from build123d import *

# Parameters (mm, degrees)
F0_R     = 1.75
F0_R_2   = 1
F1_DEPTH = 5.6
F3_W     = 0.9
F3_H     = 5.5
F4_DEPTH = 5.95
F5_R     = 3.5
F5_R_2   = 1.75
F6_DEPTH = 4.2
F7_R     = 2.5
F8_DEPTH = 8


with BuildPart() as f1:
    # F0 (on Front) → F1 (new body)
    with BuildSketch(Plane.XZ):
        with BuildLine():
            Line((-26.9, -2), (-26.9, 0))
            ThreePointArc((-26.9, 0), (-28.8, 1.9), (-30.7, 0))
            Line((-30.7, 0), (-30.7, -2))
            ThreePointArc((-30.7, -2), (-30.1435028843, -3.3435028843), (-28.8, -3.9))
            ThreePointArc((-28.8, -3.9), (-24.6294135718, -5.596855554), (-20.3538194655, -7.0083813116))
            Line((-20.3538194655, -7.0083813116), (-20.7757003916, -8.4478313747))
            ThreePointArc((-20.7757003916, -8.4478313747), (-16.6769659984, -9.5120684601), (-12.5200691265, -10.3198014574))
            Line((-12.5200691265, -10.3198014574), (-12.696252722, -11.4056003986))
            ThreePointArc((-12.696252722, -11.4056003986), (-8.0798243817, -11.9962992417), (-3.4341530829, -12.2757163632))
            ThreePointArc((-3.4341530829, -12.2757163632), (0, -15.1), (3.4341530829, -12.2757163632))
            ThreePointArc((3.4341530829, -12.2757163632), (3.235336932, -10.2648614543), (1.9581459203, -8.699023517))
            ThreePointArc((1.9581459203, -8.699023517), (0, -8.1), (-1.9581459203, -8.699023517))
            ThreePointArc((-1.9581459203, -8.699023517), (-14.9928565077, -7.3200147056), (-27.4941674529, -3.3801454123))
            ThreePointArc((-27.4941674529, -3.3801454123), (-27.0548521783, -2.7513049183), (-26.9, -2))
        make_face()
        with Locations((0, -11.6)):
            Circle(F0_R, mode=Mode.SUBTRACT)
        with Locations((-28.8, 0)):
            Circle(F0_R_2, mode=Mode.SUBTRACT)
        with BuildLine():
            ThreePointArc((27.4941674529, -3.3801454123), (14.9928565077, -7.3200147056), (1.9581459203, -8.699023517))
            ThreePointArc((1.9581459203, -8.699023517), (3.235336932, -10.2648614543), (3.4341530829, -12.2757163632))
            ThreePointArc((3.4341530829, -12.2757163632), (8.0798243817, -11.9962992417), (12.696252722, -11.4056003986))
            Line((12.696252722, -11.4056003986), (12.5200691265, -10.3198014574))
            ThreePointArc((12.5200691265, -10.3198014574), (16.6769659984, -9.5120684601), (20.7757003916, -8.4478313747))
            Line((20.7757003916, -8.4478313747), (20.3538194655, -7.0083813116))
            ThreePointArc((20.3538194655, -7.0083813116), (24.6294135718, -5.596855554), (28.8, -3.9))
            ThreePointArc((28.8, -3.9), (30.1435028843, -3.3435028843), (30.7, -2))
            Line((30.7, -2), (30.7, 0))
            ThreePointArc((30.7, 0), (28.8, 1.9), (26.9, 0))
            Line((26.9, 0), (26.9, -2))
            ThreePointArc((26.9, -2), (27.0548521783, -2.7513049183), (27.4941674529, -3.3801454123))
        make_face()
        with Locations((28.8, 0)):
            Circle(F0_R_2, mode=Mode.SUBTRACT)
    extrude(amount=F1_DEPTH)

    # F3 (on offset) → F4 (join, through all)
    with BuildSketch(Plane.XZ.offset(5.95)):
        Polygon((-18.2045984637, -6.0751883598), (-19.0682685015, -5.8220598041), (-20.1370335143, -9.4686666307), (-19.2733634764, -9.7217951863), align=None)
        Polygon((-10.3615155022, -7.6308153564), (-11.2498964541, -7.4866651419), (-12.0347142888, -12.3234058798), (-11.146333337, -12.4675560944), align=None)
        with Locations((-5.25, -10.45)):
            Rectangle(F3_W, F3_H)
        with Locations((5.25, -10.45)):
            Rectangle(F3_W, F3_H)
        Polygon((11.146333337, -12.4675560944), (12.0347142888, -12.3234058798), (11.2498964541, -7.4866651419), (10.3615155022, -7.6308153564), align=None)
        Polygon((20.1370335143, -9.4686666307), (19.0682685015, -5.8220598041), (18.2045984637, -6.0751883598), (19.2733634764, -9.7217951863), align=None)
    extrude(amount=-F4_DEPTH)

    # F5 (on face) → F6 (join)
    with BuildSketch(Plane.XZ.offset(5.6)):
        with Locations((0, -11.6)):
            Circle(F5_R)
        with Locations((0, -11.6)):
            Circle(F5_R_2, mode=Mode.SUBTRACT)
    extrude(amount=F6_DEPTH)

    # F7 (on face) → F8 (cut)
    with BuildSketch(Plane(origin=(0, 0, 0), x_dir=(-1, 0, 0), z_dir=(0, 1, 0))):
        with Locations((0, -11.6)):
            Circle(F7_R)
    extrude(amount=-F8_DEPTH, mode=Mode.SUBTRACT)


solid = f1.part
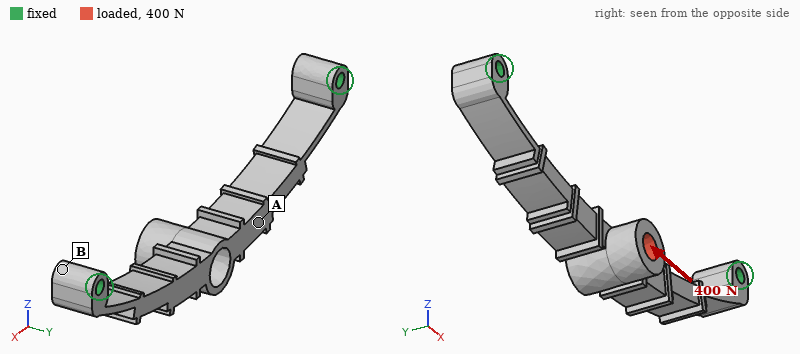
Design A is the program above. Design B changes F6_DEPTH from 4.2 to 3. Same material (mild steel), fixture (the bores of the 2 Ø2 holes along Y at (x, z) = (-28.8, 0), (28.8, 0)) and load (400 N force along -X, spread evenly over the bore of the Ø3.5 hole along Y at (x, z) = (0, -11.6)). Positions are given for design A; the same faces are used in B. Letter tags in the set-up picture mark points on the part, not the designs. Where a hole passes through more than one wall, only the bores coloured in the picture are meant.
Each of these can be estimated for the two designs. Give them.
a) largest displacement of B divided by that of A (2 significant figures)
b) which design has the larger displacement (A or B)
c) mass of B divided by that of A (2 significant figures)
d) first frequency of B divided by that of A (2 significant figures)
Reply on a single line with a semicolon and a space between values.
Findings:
0.90; A; 0.97; 1.1
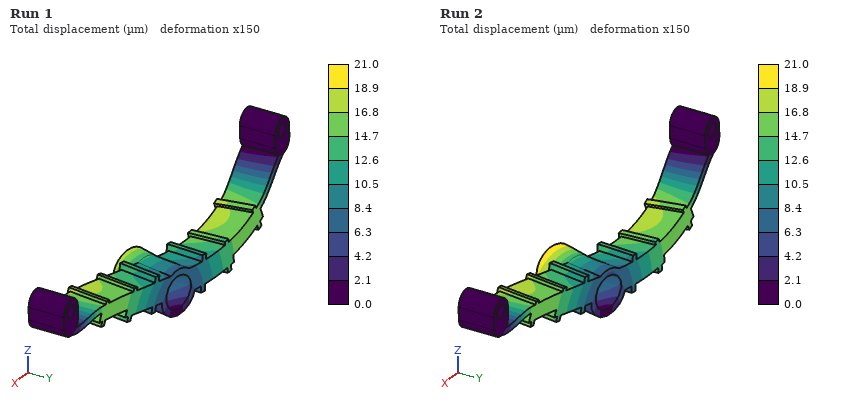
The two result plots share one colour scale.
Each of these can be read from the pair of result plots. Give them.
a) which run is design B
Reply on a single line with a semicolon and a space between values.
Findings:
Run 1
